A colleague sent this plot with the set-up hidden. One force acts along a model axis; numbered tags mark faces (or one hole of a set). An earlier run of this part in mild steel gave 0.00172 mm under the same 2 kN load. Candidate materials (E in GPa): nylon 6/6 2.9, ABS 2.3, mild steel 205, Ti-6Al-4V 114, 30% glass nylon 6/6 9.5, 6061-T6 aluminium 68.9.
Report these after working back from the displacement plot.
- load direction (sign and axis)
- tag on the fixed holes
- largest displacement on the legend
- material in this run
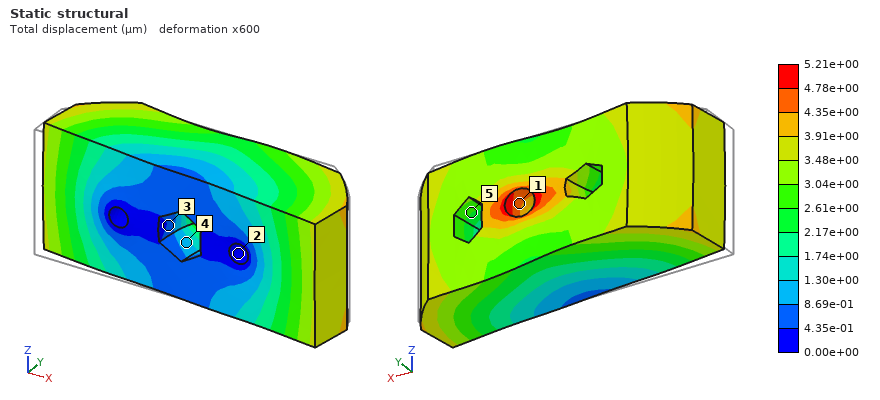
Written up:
+X
2
5.21e+00 µm
6061-T6 aluminium
